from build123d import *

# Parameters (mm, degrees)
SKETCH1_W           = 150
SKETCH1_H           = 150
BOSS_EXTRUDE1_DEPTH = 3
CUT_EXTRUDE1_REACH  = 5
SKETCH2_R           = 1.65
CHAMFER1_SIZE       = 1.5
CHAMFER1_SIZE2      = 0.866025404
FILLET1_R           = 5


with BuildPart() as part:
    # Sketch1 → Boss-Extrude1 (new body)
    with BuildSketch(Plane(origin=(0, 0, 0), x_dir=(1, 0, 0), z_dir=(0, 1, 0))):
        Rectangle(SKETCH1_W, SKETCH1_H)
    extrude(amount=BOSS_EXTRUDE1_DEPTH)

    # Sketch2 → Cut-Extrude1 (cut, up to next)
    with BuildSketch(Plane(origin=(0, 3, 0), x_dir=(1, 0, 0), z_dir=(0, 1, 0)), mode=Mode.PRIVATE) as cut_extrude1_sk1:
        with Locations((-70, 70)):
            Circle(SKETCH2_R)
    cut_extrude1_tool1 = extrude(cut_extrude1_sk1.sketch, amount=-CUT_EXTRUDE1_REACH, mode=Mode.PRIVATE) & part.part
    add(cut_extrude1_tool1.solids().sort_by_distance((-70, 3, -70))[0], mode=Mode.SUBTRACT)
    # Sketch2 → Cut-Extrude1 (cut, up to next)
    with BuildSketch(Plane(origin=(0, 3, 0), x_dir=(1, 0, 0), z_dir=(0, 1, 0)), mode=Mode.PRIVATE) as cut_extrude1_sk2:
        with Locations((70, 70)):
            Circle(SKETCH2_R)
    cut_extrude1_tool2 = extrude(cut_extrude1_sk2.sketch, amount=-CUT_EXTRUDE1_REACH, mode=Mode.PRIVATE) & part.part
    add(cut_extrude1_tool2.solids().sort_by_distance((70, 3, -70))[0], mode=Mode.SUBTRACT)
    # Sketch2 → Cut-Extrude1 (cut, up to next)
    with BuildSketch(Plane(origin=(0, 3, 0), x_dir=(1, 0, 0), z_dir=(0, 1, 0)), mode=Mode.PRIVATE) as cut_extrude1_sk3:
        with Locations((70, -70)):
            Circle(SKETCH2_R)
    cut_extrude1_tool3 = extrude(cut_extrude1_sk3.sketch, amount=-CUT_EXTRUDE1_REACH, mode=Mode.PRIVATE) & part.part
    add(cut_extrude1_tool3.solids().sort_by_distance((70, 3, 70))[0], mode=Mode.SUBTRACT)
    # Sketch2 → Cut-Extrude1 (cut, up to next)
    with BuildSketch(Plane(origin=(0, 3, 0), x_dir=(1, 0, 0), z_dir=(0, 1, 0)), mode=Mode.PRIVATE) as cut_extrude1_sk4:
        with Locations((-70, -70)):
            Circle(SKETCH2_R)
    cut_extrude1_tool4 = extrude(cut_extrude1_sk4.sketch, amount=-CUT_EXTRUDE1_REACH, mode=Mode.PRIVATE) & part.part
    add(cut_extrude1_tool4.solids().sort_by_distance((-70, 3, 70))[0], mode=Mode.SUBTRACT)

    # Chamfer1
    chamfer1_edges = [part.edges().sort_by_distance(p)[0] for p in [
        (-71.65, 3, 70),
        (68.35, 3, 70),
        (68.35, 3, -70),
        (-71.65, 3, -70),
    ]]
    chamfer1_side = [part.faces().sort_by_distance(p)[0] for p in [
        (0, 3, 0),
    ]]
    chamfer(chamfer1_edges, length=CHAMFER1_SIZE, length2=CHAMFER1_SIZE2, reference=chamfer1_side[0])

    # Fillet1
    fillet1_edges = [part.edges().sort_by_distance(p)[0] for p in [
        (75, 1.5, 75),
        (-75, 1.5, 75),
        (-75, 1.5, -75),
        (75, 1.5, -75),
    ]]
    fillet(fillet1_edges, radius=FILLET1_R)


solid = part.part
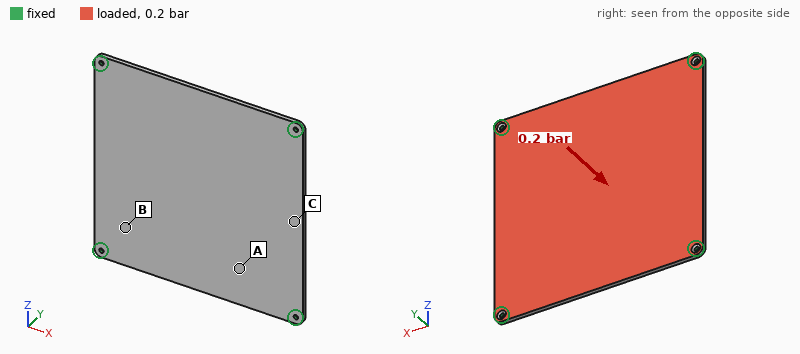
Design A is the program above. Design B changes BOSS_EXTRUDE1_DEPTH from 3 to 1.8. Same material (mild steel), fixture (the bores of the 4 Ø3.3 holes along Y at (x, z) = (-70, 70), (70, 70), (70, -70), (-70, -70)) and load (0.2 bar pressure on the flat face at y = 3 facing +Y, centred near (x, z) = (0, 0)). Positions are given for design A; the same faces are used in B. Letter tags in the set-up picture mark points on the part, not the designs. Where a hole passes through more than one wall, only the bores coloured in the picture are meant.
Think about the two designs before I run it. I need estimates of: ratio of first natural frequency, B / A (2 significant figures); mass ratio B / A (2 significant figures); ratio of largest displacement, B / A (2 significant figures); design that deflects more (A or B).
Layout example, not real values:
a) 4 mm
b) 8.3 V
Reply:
a) 0.60
b) 0.60
c) 4.6
d) B
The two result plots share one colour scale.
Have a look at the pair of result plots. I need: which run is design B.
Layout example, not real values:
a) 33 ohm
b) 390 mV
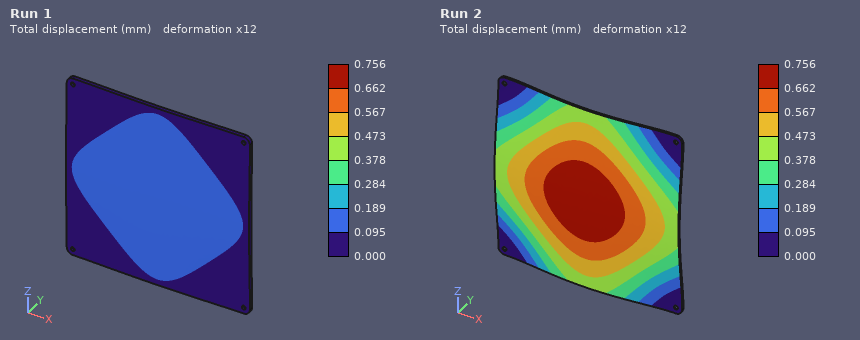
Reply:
a) Run 2
